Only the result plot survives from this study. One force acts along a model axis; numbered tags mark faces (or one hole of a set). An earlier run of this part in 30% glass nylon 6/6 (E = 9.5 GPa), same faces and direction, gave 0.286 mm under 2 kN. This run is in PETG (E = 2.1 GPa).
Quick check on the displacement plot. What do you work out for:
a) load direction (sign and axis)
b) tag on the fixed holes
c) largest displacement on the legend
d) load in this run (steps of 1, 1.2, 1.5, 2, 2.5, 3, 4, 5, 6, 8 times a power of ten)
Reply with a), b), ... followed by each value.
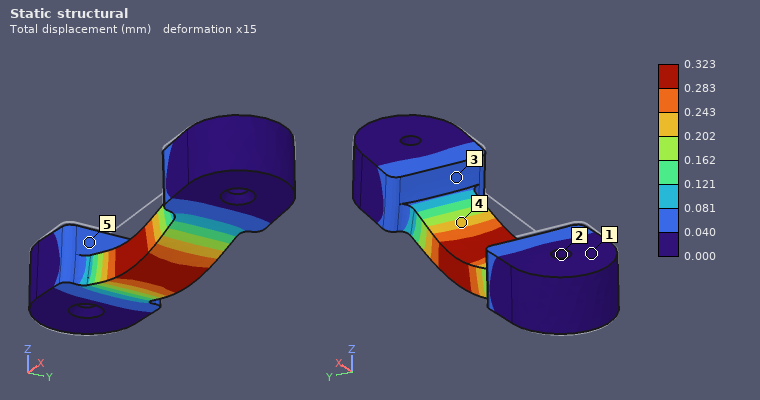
a) -Z
b) 2
c) 0.323 mm
d) 500 N
